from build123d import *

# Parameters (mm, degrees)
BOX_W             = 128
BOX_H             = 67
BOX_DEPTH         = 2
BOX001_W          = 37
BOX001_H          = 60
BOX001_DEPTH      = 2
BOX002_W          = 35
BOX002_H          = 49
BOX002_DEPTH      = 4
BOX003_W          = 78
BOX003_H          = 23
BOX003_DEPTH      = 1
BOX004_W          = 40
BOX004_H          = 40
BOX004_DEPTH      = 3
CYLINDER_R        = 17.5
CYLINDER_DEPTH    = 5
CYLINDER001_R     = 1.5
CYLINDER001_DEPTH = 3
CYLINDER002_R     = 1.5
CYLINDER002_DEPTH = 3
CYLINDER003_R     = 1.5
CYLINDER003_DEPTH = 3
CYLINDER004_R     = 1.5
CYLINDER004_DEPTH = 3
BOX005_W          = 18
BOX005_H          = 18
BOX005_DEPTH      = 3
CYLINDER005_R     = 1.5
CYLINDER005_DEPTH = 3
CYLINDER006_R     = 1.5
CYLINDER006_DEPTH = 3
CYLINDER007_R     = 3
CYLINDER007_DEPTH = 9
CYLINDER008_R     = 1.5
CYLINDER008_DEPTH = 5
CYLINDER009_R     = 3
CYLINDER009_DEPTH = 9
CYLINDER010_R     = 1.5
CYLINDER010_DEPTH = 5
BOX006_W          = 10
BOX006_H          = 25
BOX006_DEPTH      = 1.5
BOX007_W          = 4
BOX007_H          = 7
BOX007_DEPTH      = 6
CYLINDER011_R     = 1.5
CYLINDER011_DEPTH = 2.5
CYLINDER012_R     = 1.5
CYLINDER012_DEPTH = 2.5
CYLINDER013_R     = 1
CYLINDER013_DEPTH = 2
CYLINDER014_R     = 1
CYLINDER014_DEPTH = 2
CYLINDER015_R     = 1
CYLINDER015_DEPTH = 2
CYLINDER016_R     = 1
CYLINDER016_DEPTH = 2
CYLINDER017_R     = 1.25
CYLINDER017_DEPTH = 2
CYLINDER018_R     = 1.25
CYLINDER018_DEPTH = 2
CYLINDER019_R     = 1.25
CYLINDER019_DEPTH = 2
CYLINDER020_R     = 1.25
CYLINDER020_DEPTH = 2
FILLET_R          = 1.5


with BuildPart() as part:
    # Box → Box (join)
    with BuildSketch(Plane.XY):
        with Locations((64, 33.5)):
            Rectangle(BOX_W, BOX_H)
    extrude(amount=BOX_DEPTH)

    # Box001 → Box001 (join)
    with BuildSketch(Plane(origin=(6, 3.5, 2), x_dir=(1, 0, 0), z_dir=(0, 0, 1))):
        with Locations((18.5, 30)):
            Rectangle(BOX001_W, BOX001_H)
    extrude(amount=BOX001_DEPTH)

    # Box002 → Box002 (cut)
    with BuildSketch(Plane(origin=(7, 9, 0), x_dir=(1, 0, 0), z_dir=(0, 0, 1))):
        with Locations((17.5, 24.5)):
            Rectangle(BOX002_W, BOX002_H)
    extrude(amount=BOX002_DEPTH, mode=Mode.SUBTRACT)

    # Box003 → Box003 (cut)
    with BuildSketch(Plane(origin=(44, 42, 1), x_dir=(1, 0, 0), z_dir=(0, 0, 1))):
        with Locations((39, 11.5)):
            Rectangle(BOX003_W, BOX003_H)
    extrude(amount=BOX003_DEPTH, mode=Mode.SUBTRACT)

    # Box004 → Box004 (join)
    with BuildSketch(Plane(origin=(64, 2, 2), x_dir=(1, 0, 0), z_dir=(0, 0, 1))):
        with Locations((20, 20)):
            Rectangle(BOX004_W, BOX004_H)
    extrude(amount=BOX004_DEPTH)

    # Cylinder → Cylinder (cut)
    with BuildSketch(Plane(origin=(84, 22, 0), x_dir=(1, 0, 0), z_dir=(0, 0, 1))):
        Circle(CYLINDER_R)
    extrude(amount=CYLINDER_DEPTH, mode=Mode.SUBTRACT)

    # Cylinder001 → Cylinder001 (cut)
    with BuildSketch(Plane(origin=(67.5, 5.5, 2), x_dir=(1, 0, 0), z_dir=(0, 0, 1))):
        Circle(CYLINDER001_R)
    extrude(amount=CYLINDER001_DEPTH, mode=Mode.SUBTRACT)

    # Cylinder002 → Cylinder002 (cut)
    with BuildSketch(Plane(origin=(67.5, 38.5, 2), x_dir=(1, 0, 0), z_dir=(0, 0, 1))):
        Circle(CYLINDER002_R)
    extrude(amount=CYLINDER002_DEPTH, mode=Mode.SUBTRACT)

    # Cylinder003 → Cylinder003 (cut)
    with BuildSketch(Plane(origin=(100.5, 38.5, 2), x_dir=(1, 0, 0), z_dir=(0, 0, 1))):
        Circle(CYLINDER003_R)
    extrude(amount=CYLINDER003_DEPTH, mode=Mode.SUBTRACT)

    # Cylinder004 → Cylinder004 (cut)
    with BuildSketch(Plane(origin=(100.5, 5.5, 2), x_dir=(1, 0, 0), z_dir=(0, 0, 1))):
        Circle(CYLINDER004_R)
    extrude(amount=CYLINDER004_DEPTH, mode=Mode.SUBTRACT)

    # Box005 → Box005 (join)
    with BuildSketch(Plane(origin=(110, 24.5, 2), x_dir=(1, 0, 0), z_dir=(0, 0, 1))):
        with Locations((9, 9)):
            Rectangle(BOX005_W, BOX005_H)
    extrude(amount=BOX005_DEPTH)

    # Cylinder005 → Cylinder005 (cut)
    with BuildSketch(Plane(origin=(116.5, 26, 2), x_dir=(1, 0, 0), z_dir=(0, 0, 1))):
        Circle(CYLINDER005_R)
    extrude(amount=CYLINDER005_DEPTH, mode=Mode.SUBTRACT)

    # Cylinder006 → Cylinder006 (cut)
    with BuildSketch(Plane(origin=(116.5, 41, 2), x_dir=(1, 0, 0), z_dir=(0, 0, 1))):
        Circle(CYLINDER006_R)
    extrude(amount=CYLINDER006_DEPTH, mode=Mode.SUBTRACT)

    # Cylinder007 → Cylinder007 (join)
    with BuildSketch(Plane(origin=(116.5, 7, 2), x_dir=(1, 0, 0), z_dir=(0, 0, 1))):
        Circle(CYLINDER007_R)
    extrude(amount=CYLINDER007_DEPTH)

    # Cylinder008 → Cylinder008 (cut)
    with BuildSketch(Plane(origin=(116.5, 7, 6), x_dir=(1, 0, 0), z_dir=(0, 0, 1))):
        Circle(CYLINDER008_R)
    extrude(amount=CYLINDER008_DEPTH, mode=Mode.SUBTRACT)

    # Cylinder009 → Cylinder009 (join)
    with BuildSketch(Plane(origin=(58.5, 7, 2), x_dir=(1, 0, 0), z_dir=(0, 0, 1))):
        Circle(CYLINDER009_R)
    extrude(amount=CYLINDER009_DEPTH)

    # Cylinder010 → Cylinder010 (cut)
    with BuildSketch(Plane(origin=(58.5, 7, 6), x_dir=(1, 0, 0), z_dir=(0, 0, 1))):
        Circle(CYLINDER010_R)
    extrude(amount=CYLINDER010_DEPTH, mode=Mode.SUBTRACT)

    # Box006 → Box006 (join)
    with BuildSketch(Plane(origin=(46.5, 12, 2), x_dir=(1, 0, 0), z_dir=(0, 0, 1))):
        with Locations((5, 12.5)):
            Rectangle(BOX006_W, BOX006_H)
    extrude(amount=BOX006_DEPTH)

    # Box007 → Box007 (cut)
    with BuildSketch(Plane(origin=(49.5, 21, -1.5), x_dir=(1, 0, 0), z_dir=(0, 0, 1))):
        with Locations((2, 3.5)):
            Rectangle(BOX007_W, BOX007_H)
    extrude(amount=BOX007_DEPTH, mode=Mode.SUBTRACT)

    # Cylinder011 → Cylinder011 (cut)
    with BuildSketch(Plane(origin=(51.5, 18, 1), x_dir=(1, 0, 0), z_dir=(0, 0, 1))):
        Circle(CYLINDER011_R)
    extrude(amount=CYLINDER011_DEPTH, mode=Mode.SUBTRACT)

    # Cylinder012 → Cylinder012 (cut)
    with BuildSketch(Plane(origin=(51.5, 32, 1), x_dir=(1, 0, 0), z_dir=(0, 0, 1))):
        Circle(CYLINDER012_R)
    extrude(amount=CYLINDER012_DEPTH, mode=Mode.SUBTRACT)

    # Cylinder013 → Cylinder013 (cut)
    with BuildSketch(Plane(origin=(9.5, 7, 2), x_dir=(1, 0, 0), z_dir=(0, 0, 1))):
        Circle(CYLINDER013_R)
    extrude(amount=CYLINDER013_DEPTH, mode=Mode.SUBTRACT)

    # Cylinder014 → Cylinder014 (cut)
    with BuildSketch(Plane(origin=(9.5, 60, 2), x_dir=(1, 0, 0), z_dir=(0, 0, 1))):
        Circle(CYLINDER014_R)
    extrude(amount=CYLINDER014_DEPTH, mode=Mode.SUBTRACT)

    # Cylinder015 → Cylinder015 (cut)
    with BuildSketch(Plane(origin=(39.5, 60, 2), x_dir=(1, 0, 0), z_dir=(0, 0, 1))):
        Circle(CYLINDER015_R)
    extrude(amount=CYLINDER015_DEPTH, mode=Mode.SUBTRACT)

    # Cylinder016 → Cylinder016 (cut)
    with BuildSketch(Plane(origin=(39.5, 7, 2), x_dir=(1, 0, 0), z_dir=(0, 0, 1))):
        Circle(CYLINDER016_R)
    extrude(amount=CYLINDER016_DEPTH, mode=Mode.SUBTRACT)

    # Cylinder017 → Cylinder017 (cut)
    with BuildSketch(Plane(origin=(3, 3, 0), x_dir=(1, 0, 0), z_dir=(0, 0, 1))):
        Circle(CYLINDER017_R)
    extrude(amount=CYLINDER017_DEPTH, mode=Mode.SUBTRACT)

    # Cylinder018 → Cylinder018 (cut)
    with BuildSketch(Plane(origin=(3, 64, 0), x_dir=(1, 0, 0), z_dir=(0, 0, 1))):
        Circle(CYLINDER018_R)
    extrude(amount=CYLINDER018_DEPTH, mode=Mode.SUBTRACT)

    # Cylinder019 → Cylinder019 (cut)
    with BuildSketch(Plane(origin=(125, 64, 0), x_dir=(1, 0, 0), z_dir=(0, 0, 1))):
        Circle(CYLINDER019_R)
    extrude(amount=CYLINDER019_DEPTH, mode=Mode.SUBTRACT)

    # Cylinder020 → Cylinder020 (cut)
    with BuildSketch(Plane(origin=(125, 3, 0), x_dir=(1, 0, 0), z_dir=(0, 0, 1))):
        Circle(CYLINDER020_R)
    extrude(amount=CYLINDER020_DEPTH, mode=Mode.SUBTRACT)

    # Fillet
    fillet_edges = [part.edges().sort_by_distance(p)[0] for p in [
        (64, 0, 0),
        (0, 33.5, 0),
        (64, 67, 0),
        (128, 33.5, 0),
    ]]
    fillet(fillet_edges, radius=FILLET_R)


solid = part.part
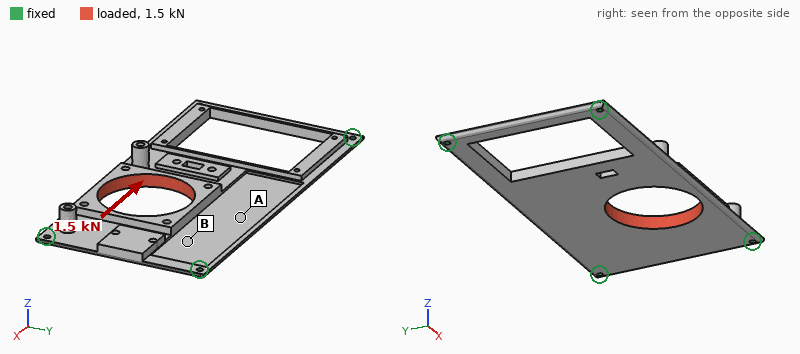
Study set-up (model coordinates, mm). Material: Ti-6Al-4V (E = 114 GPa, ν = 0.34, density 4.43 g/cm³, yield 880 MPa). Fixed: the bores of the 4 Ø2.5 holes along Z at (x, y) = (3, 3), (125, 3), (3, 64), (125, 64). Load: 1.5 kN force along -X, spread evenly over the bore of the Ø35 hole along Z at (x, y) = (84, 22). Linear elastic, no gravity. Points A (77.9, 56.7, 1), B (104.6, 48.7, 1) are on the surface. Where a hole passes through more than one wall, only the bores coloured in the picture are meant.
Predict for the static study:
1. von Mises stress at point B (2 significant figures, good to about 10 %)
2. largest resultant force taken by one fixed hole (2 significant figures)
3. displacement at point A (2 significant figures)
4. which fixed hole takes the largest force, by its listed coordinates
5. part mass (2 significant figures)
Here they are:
19 MPa
690 N
0.067 mm
(125, 3)
63 g
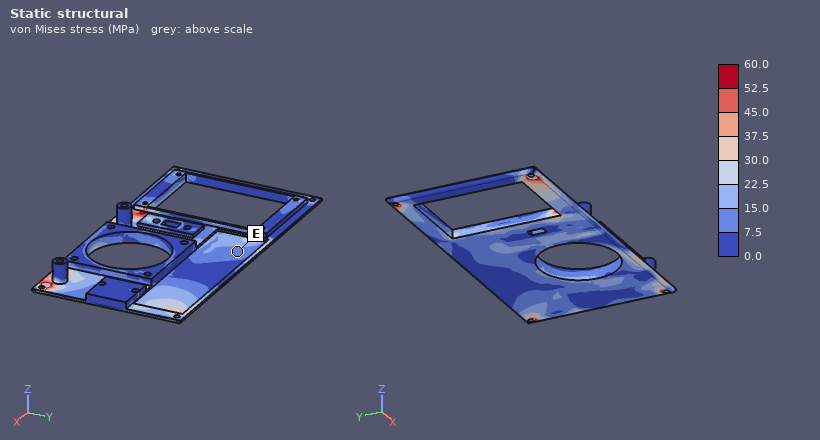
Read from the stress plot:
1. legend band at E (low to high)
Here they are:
7.5 to 15.0 MPa
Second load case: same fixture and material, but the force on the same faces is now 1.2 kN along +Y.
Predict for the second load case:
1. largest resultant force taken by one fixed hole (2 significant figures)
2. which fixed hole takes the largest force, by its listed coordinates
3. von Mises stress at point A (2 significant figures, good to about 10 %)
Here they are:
850 N
(125, 3)
25 MPa
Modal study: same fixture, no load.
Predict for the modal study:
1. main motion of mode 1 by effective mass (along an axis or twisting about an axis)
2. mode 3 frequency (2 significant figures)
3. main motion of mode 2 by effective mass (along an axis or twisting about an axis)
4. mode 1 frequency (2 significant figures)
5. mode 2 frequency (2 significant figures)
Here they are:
along Z
1700 Hz
twisting about X
600 Hz
1100 Hz
